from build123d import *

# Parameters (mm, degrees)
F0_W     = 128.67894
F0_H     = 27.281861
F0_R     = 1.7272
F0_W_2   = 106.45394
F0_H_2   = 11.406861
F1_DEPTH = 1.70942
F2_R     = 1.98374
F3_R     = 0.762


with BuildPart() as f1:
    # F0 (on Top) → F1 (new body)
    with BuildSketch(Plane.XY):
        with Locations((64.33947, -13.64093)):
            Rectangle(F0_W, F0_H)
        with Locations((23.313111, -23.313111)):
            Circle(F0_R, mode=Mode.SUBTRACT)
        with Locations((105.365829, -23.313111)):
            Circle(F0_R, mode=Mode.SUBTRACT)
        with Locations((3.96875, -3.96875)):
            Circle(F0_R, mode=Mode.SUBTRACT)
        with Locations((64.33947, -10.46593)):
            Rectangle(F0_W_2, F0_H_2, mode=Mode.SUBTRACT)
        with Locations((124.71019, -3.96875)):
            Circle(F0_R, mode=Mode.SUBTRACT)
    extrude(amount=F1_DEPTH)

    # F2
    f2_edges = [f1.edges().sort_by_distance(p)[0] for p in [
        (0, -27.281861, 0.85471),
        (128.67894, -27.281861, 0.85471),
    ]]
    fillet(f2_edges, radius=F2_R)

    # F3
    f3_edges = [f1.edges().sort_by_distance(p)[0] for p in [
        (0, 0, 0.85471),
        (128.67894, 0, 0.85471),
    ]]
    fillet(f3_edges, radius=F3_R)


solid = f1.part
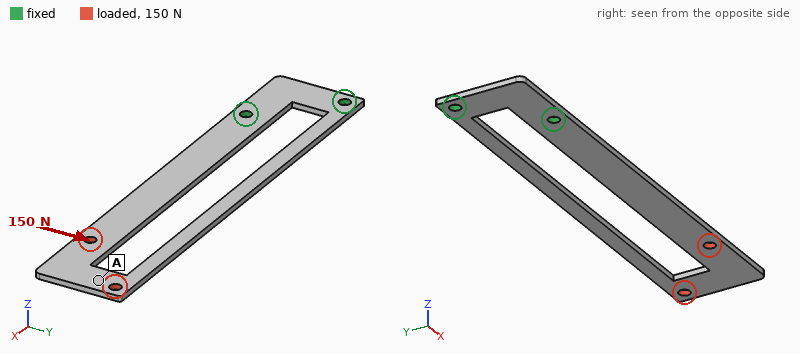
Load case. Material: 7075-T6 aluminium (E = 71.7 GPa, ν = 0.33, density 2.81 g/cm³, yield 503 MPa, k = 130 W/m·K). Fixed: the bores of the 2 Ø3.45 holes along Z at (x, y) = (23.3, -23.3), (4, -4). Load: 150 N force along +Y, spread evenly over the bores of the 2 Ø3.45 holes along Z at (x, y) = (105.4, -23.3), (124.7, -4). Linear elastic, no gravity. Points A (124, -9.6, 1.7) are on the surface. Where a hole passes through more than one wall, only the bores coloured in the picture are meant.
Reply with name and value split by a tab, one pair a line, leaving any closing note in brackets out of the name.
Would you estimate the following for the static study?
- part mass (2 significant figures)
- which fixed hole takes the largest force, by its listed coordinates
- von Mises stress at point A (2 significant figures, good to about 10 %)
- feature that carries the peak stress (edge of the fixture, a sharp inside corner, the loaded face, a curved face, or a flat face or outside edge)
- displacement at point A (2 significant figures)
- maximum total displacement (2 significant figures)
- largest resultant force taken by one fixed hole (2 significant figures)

part mass	11 g
which fixed hole takes the largest force, by its listed coordinates	(23.3, -23.3)
von Mises stress at point A	45 MPa
feature that carries the peak stress	edge of the fixture
displacement at point A	1.2 mm
maximum total displacement	1.2 mm
largest resultant force taken by one fixed hole	460 N
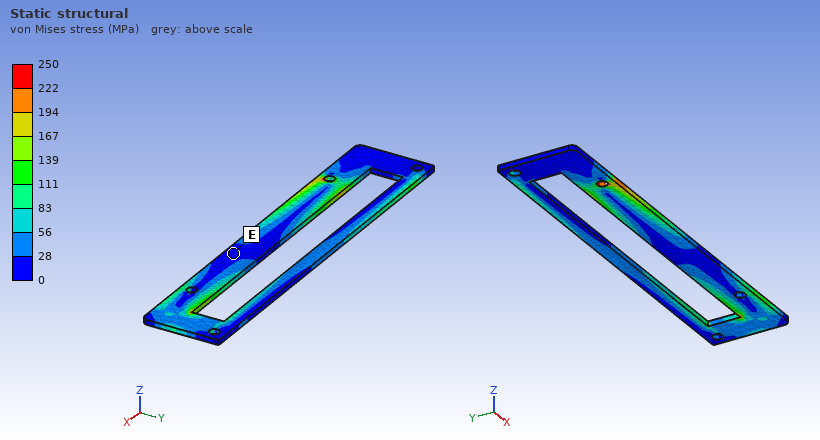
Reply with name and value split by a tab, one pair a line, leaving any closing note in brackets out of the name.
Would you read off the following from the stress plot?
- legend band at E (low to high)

legend band at E	0 to 28 MPa
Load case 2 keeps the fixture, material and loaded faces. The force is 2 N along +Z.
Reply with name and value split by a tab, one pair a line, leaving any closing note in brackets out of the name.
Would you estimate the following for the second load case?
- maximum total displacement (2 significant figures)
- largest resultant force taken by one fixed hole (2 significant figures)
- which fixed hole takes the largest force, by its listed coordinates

maximum total displacement	1.5 mm
largest resultant force taken by one fixed hole	2.1 N
which fixed hole takes the largest force, by its listed coordinates	(23.3, -23.3)
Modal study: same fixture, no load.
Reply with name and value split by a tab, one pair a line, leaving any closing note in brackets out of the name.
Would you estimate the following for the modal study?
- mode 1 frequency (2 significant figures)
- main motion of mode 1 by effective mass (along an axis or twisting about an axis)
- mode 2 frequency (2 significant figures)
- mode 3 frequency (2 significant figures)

mode 1 frequency	110 Hz
main motion of mode 1 by effective mass	along Z
mode 2 frequency	540 Hz
mode 3 frequency	700 Hz
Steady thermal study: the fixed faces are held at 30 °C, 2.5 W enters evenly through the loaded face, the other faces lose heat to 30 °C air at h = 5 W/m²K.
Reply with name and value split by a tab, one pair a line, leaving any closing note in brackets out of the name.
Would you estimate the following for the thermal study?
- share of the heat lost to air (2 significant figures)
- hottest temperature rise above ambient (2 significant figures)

share of the heat lost to air	27 %
hottest temperature rise above ambient	57 K
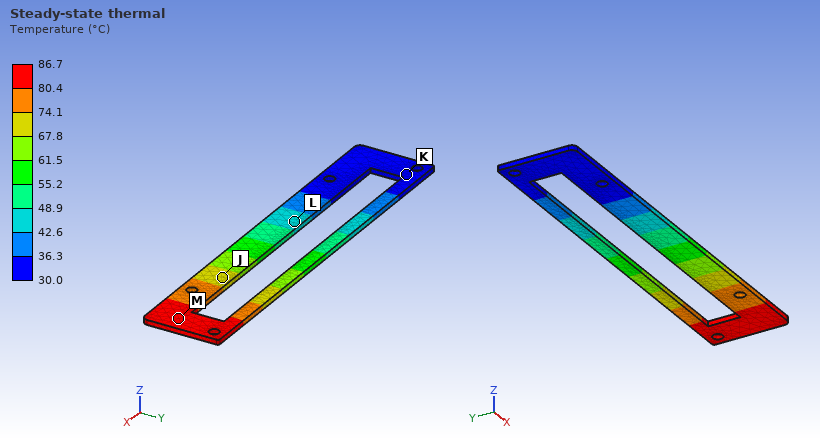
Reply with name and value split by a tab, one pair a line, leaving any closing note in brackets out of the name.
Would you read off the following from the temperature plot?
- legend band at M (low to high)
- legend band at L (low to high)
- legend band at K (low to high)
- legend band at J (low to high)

legend band at M	80.4 to 86.7 °C
legend band at L	42.6 to 48.9 °C
legend band at K	30.0 to 36.3 °C
legend band at J	67.8 to 74.1 °C
